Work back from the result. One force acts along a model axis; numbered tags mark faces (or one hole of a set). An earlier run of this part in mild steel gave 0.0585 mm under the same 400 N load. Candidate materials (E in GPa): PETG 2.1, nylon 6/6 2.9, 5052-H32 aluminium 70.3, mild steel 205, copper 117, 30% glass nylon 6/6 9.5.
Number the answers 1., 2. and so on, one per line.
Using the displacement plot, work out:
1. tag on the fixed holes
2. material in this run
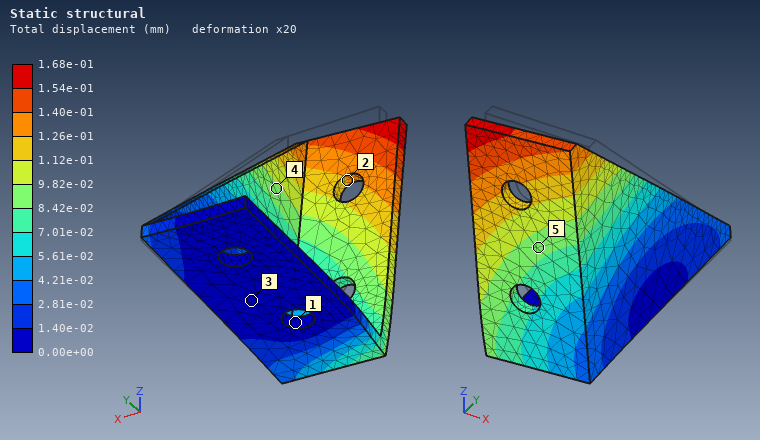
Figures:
1. 1
2. 5052-H32 aluminium
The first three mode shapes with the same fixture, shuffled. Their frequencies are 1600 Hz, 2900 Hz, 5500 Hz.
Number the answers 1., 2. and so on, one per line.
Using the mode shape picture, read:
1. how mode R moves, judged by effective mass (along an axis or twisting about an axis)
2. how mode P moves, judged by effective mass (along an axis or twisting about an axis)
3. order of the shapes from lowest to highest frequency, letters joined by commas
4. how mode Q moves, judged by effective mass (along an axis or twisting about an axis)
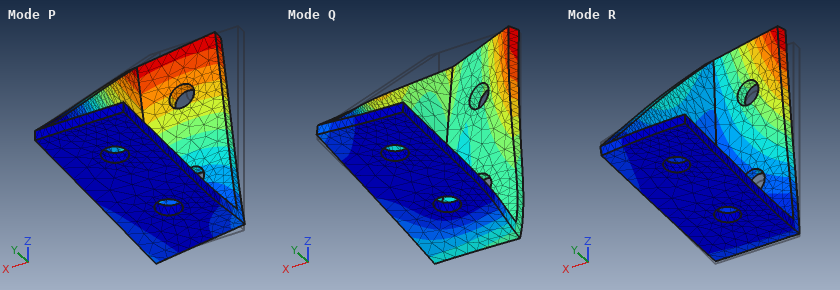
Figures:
1. along Y
2. along X
3. P, R, Q
4. along Z
